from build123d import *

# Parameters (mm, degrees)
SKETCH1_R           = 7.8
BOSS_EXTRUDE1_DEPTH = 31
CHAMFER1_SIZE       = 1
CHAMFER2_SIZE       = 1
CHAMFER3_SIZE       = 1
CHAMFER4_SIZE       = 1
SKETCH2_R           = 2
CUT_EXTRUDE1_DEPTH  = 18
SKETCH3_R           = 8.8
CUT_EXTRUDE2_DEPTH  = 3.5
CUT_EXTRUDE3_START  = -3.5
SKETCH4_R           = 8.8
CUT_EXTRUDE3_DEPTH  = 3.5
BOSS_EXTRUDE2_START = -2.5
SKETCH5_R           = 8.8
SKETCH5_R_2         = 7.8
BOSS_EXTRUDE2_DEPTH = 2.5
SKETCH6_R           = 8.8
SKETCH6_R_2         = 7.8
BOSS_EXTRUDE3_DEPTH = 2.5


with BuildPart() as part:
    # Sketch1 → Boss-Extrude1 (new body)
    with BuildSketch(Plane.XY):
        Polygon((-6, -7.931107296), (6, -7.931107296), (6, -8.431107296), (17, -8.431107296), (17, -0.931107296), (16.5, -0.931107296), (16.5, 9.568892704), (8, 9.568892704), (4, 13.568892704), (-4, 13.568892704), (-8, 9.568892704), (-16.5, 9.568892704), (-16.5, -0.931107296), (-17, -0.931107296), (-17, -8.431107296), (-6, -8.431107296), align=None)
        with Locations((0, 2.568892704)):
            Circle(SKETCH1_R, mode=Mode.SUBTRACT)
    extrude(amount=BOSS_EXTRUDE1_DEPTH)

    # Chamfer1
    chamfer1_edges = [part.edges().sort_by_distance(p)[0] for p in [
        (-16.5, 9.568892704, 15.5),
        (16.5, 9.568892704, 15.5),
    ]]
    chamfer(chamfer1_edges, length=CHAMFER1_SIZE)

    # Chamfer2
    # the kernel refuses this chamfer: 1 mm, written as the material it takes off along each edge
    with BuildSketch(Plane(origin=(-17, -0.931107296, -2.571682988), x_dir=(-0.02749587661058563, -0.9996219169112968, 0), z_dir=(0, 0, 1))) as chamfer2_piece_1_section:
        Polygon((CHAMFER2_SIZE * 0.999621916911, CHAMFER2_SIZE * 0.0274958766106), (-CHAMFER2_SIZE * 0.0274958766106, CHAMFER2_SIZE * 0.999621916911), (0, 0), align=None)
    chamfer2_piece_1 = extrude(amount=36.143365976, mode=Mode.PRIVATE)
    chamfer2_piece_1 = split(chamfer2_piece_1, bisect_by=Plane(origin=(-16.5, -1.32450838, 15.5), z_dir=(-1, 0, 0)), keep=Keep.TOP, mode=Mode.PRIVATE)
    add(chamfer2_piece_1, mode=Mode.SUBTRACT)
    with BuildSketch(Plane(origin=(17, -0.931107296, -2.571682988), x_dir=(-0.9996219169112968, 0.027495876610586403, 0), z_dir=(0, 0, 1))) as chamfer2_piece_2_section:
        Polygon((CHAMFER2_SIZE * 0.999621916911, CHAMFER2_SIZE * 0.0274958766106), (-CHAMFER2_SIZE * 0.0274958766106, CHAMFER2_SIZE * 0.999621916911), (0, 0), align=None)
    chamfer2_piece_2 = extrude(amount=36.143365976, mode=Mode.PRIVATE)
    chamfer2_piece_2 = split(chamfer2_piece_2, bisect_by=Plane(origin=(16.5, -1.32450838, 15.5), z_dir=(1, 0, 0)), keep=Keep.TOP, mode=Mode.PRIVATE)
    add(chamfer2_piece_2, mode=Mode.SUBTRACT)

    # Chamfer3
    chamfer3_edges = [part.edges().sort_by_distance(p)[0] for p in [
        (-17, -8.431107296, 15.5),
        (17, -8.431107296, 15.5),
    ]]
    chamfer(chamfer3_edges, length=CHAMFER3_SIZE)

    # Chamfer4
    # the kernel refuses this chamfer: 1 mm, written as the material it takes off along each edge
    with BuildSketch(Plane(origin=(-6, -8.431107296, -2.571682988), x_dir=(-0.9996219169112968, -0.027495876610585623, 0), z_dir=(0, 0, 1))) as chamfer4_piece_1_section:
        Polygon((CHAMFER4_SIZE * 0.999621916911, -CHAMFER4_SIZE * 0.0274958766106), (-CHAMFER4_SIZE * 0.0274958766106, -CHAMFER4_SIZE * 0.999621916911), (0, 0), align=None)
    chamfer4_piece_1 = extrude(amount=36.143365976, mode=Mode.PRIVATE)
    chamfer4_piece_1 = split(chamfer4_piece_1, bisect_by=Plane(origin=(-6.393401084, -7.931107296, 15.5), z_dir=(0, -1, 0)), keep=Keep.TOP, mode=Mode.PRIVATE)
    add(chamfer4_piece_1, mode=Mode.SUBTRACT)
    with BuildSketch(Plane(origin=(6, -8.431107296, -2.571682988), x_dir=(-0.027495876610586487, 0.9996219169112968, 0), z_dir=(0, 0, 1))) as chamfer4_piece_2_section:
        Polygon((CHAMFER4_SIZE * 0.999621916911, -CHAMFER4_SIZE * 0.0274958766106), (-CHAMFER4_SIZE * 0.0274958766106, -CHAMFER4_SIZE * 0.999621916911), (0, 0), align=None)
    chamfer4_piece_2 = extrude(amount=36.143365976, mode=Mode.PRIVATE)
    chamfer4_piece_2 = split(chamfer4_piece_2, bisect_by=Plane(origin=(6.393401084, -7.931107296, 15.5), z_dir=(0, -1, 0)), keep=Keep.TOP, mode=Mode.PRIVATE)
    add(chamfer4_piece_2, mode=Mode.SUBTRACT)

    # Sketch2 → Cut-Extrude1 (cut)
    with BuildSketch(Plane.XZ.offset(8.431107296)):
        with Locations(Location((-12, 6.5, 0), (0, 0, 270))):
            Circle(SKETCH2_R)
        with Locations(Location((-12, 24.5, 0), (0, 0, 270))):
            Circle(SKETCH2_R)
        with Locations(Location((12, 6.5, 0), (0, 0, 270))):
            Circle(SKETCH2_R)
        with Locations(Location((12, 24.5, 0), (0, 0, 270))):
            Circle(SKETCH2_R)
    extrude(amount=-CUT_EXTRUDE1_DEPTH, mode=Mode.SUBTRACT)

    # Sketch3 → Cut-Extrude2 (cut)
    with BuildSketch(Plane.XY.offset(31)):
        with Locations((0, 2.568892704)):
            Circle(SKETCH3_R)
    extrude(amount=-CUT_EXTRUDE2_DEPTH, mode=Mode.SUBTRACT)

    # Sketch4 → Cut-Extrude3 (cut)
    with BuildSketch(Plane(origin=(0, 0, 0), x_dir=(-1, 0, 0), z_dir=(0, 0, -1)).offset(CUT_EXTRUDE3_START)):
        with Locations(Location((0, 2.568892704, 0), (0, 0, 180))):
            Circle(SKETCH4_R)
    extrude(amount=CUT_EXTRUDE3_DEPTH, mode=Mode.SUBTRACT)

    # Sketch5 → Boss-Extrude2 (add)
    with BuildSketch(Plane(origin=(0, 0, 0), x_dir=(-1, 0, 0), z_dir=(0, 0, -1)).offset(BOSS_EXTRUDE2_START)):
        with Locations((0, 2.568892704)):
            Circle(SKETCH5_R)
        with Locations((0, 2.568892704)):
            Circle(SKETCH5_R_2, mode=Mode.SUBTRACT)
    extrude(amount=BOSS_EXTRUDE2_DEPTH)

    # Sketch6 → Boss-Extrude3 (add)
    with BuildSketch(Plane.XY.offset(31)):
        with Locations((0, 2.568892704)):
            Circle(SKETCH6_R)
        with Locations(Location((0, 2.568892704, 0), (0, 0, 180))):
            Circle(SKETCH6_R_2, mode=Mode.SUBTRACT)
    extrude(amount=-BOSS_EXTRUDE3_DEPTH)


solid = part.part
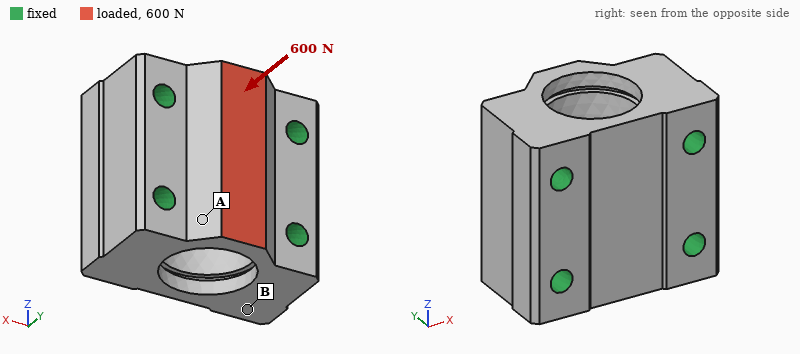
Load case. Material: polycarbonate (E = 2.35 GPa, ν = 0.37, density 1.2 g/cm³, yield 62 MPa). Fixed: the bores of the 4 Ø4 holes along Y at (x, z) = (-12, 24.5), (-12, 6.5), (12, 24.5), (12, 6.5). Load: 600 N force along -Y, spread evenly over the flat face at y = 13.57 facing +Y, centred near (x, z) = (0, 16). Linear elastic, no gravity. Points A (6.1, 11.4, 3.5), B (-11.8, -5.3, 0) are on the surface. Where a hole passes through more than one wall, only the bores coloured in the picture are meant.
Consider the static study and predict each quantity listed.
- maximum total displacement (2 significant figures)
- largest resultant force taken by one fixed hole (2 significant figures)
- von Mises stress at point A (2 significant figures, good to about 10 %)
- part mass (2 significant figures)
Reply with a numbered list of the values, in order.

1. 54 µm
2. 220 N
3. 3.5 MPa
4. 15 g
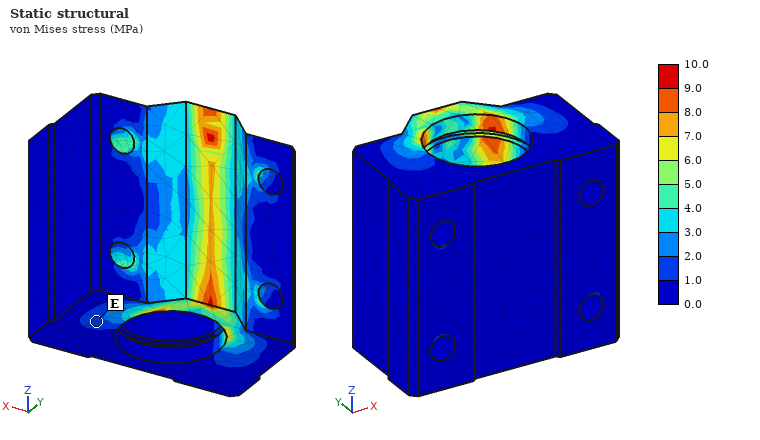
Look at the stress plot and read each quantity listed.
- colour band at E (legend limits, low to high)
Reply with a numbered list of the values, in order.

1. 1.0 to 2.0 MPa
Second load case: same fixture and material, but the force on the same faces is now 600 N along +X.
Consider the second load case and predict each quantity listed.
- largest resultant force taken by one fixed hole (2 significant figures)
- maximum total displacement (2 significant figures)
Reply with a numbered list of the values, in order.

1. 180 N
2. 24 µm
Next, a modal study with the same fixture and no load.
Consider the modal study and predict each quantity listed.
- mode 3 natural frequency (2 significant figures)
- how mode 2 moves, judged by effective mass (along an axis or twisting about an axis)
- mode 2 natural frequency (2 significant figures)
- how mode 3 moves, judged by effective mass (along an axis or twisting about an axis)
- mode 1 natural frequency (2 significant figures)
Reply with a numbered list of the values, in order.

1. 18 kHz
2. along Y
3. 16 kHz
4. along Y
5. 14 kHz
